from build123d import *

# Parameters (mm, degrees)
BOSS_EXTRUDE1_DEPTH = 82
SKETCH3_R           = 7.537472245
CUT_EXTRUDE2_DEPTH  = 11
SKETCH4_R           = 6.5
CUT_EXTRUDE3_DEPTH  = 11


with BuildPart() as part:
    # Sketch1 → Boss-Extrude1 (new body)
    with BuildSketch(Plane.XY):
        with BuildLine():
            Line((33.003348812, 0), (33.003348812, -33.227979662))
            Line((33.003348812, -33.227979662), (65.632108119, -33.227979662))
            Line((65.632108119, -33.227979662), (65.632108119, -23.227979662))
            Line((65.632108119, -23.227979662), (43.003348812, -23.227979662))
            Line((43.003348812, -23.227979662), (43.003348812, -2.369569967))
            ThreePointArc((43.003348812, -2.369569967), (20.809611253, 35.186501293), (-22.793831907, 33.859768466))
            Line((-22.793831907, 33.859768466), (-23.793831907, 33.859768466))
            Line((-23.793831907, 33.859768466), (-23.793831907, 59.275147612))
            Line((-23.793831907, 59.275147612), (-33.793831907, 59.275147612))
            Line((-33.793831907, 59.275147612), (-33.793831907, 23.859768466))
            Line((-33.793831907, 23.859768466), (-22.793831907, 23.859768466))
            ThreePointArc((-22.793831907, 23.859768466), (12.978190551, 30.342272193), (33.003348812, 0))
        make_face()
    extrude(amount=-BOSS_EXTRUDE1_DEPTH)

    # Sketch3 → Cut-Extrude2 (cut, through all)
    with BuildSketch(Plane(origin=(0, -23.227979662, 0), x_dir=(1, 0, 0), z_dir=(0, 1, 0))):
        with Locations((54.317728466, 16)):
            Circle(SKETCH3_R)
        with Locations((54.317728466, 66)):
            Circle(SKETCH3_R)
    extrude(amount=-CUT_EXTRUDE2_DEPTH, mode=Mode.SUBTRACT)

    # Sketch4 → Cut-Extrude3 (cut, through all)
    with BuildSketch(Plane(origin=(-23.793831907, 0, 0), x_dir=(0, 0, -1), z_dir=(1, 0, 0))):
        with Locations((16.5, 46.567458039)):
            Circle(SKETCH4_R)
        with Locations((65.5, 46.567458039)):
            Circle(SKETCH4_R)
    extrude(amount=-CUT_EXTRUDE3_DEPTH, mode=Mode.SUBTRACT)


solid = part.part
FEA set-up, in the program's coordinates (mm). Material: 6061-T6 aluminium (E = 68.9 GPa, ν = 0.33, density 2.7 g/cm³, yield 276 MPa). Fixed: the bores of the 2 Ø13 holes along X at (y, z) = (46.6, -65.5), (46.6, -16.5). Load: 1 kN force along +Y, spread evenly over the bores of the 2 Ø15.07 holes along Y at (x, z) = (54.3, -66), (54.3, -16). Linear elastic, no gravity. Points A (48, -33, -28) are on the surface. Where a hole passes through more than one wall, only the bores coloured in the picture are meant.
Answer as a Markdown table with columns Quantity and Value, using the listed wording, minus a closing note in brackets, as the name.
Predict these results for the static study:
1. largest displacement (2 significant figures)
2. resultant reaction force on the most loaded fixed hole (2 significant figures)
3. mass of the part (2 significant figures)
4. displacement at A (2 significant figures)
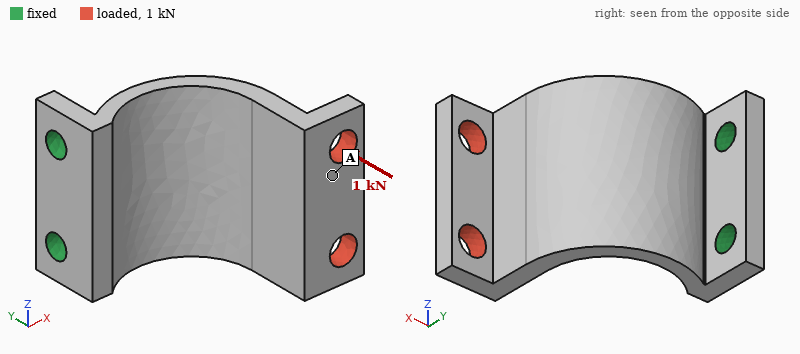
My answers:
| Quantity | Value |
|---|---|
| largest displacement | 1.6 mm |
| resultant reaction force on the most loaded fixed hole | 510 N |
| mass of the part | 340 g |
| displacement at A | 1.4 mm |
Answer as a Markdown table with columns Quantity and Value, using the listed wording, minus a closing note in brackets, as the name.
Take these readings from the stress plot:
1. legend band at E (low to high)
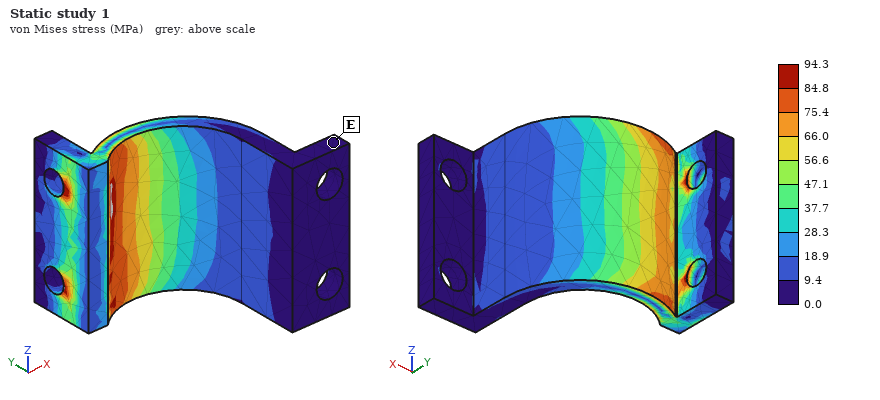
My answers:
| Quantity | Value |
|---|---|
| legend band at E | 0.0 to 9.4 MPa |
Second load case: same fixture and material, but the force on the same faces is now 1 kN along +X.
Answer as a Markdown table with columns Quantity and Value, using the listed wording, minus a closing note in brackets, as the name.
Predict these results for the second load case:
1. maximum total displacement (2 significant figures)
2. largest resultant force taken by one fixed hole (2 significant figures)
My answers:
| Quantity | Value |
|---|---|
| maximum total displacement | 1.8 mm |
| largest resultant force taken by one fixed hole | 500 N |
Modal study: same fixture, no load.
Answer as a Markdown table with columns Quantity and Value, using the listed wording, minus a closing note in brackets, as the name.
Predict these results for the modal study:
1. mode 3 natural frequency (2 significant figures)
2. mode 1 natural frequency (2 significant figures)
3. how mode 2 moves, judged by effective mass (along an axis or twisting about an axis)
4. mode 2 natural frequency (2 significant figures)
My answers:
| Quantity | Value |
|---|---|
| mode 3 natural frequency | 1400 Hz |
| mode 1 natural frequency | 340 Hz |
| how mode 2 moves, judged by effective mass | along Z |
| mode 2 natural frequency | 720 Hz |
